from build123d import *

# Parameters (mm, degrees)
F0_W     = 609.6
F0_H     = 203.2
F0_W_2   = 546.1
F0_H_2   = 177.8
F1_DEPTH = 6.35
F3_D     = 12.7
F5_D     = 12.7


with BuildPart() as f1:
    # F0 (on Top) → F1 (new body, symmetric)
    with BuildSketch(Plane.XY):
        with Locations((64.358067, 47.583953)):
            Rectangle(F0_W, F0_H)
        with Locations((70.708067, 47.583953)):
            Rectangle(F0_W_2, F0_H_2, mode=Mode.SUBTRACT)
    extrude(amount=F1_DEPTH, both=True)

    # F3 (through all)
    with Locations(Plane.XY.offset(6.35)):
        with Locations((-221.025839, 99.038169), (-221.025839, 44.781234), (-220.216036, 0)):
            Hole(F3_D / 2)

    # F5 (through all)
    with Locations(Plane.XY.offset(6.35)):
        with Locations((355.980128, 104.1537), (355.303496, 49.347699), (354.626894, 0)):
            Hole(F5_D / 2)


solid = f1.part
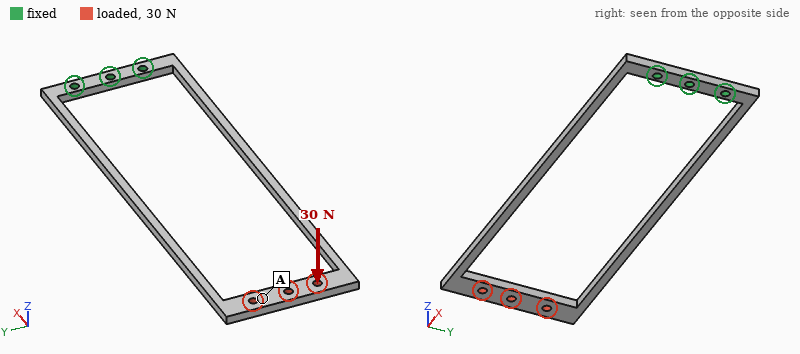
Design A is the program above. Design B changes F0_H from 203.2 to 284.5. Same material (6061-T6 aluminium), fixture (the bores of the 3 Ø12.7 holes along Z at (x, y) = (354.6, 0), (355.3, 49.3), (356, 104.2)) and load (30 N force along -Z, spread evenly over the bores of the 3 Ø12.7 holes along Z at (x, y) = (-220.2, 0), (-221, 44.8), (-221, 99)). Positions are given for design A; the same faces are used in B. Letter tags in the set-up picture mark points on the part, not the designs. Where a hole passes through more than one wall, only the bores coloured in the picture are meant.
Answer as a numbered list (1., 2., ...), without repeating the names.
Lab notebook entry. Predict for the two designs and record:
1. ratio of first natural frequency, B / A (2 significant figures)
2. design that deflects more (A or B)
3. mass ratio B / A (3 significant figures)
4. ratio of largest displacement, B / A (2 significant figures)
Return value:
1. 1.2
2. A
3. 2.91
4. 0.32
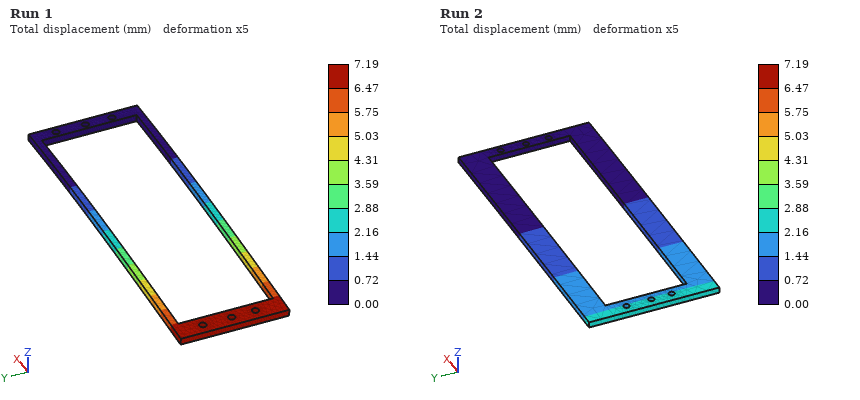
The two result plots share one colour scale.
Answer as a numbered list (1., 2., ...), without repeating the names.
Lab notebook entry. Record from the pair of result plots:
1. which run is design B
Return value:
1. Run 2
